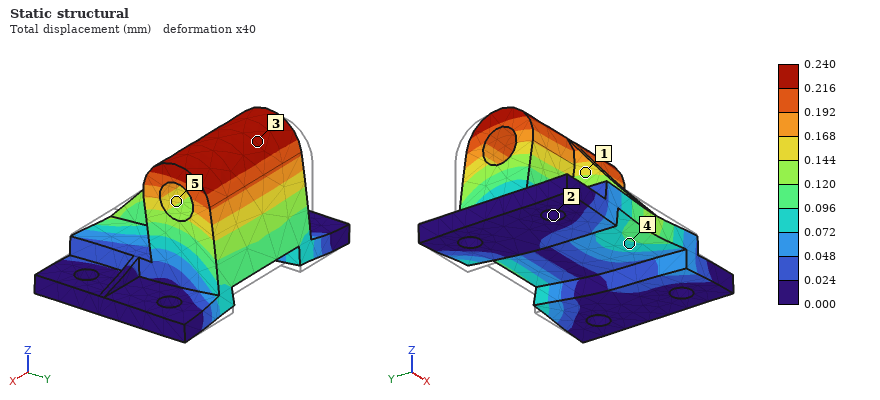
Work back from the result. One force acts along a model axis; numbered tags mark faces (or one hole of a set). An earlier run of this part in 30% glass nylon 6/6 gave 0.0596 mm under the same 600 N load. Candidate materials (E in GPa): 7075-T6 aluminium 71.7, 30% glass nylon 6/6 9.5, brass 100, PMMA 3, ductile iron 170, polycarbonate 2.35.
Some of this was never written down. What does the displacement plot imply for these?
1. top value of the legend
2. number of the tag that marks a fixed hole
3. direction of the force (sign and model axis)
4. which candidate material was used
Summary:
0.240 mm
2
-Y
polycarbonate
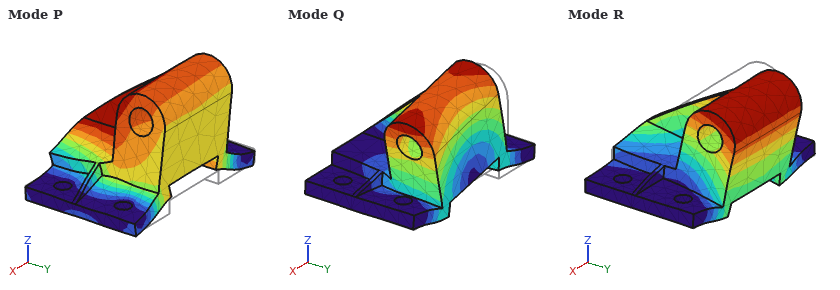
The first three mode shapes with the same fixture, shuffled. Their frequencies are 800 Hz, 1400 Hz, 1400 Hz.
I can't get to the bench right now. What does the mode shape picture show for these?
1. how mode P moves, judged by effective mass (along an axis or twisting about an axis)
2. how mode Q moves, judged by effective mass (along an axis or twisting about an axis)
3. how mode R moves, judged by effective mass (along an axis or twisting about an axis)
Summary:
along Z
along X
along Y
